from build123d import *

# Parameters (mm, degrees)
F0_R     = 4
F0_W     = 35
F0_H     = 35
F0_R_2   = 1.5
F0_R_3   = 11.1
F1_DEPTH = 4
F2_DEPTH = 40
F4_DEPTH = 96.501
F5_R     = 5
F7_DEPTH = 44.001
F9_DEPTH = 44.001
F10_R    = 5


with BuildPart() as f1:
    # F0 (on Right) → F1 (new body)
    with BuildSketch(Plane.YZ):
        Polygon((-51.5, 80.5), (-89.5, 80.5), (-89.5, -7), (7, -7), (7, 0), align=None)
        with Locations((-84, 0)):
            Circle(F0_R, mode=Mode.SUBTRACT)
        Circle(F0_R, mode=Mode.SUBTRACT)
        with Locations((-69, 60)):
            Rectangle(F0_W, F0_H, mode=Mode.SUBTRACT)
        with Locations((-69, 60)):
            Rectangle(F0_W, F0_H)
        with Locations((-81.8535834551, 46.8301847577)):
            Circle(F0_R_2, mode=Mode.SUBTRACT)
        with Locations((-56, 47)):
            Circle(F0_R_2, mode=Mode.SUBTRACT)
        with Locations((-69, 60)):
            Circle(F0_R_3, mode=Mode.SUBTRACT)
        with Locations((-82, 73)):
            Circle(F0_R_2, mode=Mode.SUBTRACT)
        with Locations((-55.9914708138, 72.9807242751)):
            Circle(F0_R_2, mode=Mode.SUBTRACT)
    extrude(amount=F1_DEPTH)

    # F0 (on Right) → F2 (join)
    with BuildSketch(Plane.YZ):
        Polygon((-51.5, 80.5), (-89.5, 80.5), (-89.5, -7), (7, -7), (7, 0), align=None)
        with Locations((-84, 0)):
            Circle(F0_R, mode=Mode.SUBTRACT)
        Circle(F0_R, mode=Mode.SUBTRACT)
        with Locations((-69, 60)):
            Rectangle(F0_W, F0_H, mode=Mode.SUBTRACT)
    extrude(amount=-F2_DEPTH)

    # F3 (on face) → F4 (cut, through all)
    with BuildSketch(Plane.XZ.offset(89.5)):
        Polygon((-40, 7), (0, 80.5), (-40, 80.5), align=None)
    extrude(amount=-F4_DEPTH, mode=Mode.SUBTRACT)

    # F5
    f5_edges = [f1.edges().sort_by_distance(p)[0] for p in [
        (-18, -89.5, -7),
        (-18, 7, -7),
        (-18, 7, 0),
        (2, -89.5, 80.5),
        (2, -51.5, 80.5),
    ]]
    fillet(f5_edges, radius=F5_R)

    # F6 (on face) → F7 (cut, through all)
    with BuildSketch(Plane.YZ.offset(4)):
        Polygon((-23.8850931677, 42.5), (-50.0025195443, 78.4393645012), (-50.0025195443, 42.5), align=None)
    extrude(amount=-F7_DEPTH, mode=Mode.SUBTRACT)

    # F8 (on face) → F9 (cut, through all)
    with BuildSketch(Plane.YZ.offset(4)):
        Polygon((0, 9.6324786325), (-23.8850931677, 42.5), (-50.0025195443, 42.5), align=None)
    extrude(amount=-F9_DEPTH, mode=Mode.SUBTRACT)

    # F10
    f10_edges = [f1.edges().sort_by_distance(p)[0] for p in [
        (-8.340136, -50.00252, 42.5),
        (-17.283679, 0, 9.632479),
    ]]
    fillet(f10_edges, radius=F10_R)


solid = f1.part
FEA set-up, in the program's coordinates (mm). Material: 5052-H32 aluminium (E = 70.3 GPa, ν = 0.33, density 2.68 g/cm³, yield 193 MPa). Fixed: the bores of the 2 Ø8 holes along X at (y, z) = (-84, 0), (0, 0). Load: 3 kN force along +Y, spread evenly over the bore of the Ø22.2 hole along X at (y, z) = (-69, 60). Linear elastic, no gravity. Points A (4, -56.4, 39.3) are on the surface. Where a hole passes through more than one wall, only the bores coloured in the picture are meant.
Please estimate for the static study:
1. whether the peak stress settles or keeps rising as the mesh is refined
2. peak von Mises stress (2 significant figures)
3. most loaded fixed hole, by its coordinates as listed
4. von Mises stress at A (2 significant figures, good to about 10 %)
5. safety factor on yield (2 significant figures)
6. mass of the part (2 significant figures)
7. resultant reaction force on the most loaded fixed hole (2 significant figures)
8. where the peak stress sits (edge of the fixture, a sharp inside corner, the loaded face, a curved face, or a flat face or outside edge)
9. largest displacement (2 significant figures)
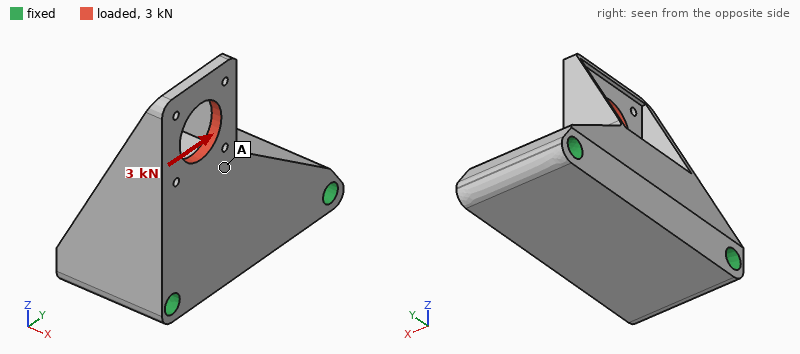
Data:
settles
130 MPa
(0, 0)
14 MPa
1.5
390 g
3.3 kN
the loaded face
0.10 mm
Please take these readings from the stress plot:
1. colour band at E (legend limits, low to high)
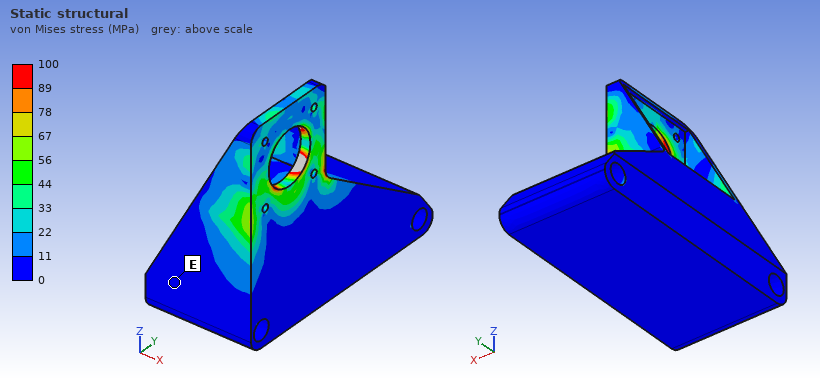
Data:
0 to 11 MPa
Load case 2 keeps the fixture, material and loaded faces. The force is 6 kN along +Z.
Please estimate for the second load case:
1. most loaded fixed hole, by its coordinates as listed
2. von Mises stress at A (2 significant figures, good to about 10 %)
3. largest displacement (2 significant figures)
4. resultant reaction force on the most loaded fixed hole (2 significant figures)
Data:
(-84, 0)
31 MPa
78 µm
5.1 kN
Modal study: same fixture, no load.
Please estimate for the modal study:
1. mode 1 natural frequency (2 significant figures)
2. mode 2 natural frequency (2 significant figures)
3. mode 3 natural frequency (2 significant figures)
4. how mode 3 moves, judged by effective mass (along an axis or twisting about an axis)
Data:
5500 Hz
7100 Hz
9400 Hz
along X
